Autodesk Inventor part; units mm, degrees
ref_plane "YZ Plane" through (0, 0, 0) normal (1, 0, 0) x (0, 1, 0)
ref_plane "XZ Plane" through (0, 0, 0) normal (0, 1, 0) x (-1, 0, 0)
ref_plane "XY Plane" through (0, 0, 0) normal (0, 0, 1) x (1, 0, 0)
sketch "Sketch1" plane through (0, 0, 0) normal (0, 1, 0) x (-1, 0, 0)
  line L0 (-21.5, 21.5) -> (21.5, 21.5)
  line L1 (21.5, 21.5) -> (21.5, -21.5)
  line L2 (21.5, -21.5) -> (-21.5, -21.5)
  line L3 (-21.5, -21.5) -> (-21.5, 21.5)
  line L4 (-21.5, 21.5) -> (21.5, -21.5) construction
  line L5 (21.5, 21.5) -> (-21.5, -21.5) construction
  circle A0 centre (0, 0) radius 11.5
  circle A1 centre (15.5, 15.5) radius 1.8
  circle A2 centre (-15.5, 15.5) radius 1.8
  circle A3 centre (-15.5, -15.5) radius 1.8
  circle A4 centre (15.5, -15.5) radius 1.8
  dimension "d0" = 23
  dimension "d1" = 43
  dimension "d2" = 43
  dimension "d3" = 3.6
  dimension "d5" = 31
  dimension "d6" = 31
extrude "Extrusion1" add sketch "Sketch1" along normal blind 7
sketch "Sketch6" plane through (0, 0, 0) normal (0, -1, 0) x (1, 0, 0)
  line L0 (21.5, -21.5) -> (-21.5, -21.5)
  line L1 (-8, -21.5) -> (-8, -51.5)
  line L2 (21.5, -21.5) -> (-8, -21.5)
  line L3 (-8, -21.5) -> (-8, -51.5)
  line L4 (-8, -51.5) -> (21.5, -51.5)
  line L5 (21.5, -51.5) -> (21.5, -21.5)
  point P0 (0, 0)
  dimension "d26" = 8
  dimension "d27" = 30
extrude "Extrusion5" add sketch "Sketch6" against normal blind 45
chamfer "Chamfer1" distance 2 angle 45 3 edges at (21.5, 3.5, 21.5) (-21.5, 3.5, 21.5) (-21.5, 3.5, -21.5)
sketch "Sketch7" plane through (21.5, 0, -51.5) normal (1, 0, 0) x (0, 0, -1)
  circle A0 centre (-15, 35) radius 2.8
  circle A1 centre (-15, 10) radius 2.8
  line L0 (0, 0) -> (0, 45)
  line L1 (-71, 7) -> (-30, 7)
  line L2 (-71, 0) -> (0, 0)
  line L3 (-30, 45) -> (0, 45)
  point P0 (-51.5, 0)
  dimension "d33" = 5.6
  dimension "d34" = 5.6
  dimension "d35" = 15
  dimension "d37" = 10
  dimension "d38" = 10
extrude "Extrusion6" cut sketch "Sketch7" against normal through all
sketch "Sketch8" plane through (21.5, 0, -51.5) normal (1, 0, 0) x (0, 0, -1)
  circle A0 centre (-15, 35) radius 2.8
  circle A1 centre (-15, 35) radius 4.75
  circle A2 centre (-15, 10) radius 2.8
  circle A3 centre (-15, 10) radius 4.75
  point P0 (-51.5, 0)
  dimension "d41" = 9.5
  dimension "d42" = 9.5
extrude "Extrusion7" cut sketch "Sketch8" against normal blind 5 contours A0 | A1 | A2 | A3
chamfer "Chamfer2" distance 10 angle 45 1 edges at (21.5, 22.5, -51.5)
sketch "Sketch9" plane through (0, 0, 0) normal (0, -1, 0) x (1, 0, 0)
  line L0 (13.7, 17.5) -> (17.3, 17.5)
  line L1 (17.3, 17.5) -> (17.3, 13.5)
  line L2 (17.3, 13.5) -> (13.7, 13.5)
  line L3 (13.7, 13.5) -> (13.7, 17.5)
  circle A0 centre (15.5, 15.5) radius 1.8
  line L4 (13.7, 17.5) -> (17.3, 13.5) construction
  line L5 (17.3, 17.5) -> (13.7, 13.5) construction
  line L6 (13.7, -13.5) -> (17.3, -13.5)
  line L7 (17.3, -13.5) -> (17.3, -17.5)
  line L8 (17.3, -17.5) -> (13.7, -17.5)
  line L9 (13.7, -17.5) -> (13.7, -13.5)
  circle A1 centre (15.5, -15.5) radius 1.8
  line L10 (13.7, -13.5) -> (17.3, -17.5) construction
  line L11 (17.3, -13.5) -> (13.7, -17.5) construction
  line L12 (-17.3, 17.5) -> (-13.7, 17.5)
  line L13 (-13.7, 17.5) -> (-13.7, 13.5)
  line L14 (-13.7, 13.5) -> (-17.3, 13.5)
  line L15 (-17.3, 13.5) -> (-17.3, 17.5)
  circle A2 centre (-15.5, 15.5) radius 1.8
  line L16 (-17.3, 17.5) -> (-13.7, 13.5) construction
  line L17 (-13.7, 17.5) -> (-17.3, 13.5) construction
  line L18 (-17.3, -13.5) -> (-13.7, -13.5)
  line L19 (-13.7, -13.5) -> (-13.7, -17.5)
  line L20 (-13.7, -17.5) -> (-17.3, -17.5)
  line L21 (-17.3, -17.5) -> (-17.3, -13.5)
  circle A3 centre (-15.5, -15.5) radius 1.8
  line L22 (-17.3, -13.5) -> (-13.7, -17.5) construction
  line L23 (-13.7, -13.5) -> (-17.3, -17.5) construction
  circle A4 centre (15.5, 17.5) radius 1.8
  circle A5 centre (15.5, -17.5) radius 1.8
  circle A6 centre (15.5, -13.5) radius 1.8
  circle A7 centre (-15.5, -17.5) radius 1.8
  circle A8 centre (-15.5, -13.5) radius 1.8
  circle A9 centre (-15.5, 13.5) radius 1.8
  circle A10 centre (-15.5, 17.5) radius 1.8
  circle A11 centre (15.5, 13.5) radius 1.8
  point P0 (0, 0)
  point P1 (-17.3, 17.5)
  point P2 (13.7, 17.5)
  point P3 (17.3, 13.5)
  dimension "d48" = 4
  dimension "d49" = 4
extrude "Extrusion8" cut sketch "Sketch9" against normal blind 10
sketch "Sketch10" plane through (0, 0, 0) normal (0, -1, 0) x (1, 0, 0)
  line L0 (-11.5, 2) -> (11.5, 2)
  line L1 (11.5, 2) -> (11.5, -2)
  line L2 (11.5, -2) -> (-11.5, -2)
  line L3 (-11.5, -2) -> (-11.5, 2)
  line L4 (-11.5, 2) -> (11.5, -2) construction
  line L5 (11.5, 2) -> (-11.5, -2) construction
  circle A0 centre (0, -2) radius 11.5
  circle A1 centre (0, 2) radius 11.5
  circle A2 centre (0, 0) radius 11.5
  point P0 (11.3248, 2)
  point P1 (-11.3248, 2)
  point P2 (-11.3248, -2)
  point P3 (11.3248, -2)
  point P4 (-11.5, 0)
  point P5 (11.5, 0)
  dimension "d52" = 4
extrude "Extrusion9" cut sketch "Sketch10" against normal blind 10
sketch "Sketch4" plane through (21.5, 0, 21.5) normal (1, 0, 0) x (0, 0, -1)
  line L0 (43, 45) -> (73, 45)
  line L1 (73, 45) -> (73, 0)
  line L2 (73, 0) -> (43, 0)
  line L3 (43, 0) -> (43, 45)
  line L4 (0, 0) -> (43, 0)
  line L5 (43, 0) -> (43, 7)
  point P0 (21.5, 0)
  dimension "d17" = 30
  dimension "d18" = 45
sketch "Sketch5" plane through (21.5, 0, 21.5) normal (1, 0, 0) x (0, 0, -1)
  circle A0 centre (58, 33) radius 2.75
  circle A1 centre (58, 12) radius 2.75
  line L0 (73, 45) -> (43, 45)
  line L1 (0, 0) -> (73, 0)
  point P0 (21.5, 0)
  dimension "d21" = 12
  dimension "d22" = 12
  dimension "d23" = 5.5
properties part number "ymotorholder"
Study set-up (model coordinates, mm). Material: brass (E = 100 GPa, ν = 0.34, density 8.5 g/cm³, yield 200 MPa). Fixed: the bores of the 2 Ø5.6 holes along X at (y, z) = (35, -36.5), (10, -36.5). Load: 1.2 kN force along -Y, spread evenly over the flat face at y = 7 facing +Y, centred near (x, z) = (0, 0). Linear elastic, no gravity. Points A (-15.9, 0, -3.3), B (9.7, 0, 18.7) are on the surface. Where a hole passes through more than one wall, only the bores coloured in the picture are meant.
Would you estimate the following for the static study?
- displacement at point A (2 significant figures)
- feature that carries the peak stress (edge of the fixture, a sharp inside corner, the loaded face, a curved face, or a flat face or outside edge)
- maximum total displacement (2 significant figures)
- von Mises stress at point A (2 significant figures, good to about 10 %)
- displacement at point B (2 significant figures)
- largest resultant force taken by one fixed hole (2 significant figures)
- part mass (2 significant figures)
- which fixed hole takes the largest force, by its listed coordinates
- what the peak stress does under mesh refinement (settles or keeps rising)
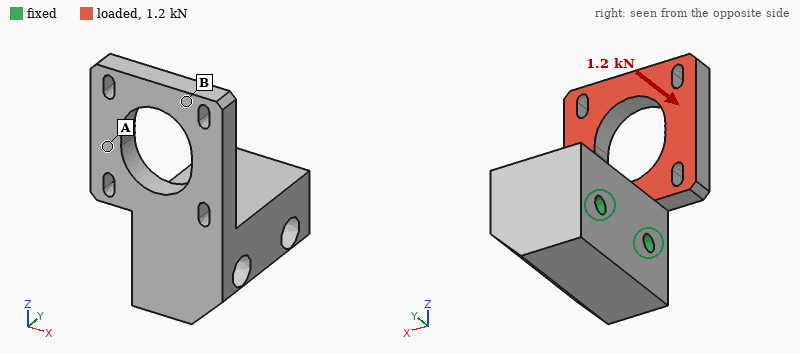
0.12 mm
a sharp inside corner
0.33 mm
43 MPa
0.25 mm
1.7 kN
380 g
(35, -36.5)
keeps rising
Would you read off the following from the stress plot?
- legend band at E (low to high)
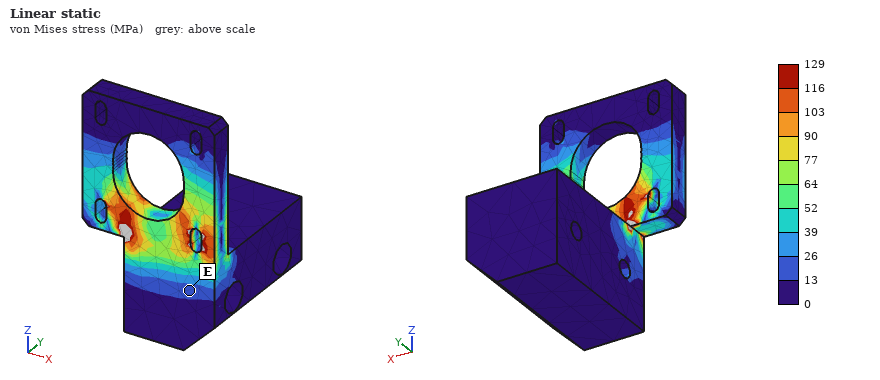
13 to 26 MPa
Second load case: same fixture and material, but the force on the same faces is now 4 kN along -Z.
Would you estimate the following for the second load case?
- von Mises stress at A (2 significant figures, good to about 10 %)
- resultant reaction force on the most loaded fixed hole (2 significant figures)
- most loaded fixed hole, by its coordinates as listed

25 MPa
4.3 kN
(10, -36.5)
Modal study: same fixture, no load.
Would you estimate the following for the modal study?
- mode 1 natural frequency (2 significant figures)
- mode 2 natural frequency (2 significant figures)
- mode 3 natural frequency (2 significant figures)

1400 Hz
2900 Hz
3100 Hz
